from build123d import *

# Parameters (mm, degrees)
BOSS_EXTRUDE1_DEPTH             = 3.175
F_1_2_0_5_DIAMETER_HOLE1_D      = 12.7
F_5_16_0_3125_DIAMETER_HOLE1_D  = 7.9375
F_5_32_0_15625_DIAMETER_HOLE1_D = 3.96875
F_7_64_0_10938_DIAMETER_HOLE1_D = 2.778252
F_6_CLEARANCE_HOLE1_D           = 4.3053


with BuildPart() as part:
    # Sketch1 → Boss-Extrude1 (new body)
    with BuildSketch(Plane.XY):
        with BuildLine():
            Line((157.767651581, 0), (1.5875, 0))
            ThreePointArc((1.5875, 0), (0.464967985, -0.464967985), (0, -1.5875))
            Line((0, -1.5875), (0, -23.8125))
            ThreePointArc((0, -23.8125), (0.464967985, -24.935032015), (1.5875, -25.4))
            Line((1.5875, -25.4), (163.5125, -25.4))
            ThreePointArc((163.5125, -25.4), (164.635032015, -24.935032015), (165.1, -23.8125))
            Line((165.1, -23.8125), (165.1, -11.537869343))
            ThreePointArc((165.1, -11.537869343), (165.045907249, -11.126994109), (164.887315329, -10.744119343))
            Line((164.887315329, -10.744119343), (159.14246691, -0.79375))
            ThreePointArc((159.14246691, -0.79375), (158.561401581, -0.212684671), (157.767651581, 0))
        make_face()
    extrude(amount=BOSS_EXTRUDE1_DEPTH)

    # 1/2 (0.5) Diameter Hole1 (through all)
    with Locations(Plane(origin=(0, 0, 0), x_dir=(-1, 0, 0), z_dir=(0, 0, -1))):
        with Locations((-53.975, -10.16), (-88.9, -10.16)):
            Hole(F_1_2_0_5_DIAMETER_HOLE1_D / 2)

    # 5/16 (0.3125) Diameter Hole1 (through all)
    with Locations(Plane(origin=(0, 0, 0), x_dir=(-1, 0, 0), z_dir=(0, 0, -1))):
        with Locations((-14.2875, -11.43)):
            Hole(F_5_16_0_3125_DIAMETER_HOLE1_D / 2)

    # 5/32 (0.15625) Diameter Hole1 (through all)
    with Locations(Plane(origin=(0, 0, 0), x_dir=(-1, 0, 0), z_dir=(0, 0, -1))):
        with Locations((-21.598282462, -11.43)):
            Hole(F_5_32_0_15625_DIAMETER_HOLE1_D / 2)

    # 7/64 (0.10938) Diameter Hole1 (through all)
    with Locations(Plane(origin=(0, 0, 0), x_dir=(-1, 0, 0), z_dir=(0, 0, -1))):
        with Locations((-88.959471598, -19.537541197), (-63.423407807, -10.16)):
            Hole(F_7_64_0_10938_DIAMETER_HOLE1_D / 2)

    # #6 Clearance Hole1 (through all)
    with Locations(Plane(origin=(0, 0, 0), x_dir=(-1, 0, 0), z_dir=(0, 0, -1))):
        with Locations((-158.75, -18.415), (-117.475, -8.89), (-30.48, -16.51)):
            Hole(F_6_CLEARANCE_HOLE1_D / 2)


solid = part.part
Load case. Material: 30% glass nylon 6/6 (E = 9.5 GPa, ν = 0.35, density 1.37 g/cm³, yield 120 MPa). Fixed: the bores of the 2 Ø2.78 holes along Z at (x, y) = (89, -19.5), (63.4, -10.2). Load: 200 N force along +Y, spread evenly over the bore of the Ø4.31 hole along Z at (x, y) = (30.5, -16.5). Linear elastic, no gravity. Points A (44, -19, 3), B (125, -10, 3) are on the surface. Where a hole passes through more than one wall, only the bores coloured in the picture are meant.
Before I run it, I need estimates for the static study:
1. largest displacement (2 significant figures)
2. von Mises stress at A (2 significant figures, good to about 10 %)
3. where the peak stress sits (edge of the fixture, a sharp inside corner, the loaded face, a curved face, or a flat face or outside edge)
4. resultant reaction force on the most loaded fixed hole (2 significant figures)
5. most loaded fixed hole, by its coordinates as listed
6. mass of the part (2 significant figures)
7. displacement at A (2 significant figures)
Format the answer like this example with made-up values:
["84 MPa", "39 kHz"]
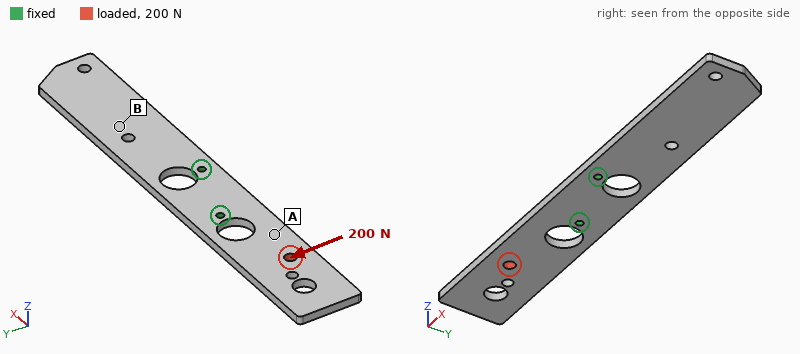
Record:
["0.42 mm", "4.9 MPa", "edge of the fixture", "410 N", "(63.4, -10.2)", "16 g", "0.14 mm"]
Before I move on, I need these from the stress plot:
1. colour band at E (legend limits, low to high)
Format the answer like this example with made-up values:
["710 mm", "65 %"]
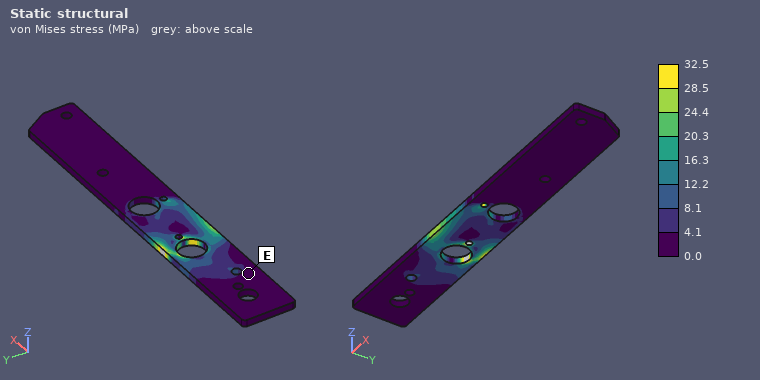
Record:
["0.0 to 4.1 MPa"]
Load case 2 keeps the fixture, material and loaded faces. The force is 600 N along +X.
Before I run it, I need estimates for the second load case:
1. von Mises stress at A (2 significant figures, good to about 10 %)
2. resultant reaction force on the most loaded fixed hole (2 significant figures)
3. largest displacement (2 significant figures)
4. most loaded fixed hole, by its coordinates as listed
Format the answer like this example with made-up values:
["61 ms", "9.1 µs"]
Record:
["14 MPa", "350 N", "0.15 mm", "(63.4, -10.2)"]
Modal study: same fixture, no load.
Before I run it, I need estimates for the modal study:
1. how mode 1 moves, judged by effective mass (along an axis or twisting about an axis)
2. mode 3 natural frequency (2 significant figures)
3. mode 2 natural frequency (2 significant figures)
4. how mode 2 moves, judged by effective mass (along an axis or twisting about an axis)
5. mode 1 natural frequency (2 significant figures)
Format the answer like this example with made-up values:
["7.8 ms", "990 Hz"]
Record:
["along Z", "1100 Hz", "260 Hz", "along Z", "210 Hz"]
